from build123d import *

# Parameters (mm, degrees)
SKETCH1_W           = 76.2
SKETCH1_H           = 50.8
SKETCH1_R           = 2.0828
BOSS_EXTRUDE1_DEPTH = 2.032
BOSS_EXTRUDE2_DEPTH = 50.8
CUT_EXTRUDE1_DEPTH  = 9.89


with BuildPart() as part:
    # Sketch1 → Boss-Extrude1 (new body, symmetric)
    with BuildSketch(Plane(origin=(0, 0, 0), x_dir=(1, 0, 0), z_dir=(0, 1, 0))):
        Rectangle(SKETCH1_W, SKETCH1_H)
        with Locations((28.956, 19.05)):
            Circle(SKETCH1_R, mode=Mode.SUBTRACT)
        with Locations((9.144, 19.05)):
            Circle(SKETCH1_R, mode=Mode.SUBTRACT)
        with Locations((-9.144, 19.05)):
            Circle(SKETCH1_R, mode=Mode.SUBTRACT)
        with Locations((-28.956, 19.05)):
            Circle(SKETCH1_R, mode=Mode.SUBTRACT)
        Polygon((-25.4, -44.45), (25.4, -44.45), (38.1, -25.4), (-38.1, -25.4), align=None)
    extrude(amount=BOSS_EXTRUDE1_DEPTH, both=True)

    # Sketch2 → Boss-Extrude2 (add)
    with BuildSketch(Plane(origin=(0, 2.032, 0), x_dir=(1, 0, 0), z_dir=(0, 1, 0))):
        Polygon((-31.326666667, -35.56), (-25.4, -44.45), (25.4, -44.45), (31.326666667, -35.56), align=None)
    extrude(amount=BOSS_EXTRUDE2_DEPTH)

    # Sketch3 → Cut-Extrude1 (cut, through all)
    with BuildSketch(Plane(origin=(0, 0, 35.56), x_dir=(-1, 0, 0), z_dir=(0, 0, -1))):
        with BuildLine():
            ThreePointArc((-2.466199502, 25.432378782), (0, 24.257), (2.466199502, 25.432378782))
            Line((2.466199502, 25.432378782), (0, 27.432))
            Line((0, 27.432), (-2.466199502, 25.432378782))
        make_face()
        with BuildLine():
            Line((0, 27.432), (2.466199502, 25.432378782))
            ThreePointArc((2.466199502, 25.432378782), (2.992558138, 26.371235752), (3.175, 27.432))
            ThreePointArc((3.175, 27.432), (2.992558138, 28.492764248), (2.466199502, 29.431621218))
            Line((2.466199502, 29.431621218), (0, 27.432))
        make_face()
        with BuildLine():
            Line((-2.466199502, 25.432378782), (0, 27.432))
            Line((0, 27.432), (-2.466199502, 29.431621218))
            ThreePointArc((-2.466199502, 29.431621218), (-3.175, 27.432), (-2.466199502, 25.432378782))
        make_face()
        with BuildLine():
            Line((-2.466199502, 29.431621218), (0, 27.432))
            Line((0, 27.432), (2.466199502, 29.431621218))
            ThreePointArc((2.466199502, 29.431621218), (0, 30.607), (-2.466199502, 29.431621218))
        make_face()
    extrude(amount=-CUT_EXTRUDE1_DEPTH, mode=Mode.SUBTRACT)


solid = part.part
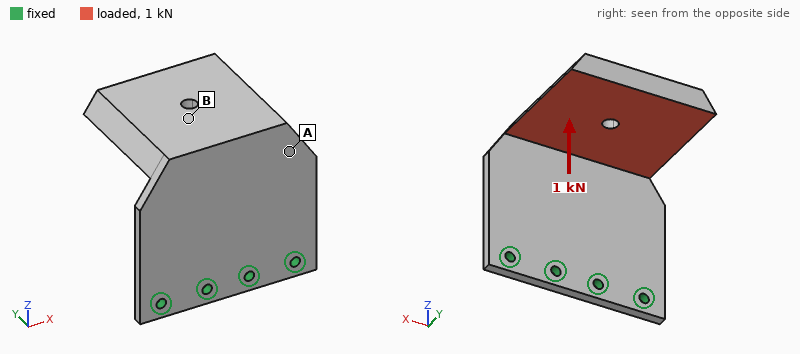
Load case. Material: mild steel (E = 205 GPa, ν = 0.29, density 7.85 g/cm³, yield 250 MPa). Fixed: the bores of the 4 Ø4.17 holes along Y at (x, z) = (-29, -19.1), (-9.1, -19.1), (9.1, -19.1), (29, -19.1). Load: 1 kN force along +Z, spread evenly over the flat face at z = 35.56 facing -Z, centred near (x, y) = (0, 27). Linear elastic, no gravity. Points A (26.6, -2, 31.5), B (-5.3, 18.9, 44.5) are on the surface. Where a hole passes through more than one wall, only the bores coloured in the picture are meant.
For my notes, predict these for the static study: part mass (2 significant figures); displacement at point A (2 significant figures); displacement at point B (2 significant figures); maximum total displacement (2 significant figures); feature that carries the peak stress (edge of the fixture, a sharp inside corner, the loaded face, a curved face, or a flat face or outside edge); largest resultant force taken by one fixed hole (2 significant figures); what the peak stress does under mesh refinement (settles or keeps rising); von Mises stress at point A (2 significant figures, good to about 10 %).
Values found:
360 g
0.38 mm
0.69 mm
1.1 mm
edge of the fixture
260 N
keeps rising
140 MPa
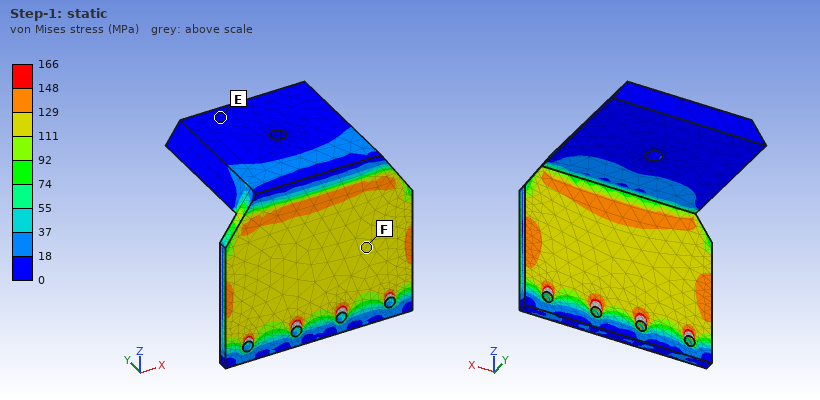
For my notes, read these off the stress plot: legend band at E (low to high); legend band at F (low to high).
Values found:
0 to 18 MPa
111 to 129 MPa
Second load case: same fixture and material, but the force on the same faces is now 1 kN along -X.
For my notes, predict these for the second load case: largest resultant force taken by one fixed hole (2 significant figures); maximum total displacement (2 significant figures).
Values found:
970 N
0.38 mm
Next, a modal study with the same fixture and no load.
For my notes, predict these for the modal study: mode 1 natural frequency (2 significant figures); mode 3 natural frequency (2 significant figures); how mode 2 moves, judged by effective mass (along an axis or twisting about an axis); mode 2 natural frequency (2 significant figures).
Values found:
300 Hz
1100 Hz
along X
650 Hz
